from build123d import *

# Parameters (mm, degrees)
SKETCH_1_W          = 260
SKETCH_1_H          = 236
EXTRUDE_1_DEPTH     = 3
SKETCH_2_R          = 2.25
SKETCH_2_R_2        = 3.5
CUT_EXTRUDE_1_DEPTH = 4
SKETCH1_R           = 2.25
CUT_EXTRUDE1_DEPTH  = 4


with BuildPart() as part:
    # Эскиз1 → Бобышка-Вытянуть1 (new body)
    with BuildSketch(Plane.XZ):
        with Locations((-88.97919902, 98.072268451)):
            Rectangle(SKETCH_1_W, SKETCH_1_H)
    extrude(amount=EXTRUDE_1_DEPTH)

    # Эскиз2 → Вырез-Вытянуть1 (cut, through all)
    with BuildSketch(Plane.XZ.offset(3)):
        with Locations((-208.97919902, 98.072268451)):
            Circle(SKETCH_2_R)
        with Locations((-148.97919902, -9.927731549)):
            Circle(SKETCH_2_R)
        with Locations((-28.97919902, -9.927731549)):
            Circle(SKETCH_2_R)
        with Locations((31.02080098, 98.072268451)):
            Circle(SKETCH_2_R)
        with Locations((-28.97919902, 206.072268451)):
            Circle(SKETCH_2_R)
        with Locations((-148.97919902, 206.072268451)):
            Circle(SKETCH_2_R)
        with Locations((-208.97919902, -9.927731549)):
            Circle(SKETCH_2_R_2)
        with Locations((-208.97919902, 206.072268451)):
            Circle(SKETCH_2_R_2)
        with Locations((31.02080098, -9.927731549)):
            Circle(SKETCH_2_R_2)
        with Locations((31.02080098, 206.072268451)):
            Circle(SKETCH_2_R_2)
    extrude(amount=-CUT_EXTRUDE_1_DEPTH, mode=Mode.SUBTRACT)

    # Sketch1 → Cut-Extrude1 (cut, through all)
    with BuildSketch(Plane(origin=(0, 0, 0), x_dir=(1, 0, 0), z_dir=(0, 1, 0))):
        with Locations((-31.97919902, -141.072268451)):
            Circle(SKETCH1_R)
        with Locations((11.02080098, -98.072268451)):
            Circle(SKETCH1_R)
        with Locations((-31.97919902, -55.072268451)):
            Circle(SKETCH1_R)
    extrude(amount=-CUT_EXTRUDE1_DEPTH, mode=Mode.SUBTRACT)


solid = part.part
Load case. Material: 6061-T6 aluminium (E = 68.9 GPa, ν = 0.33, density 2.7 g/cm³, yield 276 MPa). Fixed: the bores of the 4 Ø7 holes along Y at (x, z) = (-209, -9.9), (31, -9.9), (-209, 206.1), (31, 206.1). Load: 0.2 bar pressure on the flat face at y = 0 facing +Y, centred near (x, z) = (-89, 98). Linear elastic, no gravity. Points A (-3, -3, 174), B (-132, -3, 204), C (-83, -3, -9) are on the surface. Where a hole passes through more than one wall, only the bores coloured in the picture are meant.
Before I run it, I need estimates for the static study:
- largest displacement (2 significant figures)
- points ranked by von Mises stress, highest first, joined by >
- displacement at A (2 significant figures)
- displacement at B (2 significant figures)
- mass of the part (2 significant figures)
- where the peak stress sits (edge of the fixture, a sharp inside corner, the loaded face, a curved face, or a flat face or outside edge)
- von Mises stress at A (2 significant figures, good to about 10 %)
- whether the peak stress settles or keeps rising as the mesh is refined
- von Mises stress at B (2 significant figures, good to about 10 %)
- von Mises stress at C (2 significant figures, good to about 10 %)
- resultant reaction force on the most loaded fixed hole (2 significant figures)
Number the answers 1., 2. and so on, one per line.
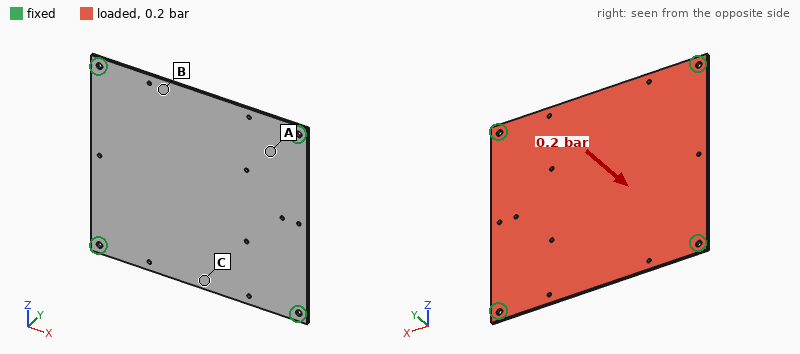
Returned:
1. 2.8 mm
2. C > B > A
3. 0.99 mm
4. 1.5 mm
5. 490 g
6. edge of the fixture
7. 13 MPa
8. keeps rising
9. 36 MPa
10. 49 MPa
11. 310 N
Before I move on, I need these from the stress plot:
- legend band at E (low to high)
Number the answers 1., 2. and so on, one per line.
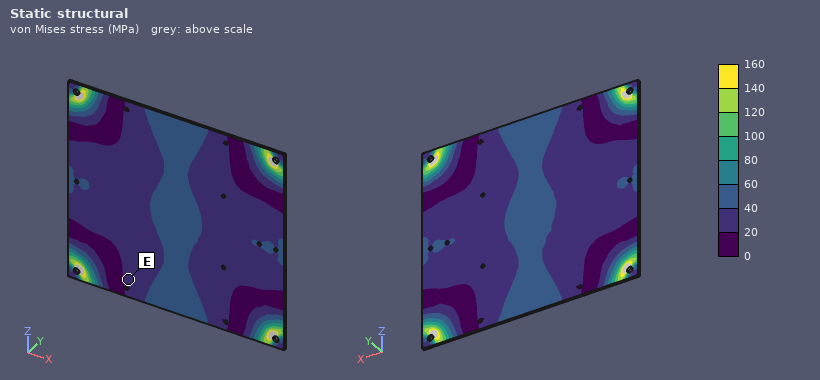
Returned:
1. 20 to 40 MPa
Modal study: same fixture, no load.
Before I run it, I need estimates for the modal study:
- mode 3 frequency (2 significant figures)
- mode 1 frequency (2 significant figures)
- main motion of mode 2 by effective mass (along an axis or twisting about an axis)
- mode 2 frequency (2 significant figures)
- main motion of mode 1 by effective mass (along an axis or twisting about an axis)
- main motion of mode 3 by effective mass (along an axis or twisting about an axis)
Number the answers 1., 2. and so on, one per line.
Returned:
1. 350 Hz
2. 180 Hz
3. twisting about X
4. 310 Hz
5. along Y
6. twisting about Z
